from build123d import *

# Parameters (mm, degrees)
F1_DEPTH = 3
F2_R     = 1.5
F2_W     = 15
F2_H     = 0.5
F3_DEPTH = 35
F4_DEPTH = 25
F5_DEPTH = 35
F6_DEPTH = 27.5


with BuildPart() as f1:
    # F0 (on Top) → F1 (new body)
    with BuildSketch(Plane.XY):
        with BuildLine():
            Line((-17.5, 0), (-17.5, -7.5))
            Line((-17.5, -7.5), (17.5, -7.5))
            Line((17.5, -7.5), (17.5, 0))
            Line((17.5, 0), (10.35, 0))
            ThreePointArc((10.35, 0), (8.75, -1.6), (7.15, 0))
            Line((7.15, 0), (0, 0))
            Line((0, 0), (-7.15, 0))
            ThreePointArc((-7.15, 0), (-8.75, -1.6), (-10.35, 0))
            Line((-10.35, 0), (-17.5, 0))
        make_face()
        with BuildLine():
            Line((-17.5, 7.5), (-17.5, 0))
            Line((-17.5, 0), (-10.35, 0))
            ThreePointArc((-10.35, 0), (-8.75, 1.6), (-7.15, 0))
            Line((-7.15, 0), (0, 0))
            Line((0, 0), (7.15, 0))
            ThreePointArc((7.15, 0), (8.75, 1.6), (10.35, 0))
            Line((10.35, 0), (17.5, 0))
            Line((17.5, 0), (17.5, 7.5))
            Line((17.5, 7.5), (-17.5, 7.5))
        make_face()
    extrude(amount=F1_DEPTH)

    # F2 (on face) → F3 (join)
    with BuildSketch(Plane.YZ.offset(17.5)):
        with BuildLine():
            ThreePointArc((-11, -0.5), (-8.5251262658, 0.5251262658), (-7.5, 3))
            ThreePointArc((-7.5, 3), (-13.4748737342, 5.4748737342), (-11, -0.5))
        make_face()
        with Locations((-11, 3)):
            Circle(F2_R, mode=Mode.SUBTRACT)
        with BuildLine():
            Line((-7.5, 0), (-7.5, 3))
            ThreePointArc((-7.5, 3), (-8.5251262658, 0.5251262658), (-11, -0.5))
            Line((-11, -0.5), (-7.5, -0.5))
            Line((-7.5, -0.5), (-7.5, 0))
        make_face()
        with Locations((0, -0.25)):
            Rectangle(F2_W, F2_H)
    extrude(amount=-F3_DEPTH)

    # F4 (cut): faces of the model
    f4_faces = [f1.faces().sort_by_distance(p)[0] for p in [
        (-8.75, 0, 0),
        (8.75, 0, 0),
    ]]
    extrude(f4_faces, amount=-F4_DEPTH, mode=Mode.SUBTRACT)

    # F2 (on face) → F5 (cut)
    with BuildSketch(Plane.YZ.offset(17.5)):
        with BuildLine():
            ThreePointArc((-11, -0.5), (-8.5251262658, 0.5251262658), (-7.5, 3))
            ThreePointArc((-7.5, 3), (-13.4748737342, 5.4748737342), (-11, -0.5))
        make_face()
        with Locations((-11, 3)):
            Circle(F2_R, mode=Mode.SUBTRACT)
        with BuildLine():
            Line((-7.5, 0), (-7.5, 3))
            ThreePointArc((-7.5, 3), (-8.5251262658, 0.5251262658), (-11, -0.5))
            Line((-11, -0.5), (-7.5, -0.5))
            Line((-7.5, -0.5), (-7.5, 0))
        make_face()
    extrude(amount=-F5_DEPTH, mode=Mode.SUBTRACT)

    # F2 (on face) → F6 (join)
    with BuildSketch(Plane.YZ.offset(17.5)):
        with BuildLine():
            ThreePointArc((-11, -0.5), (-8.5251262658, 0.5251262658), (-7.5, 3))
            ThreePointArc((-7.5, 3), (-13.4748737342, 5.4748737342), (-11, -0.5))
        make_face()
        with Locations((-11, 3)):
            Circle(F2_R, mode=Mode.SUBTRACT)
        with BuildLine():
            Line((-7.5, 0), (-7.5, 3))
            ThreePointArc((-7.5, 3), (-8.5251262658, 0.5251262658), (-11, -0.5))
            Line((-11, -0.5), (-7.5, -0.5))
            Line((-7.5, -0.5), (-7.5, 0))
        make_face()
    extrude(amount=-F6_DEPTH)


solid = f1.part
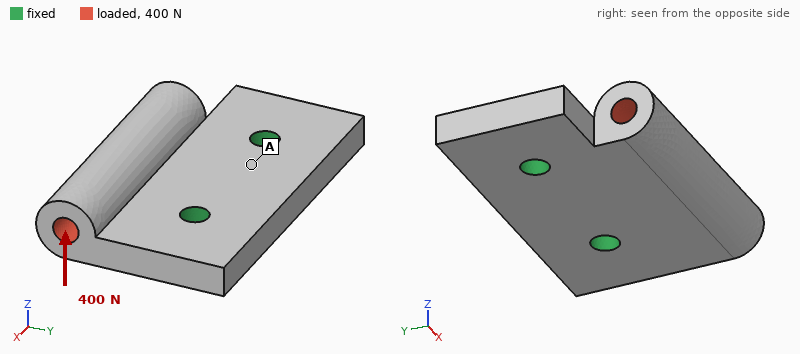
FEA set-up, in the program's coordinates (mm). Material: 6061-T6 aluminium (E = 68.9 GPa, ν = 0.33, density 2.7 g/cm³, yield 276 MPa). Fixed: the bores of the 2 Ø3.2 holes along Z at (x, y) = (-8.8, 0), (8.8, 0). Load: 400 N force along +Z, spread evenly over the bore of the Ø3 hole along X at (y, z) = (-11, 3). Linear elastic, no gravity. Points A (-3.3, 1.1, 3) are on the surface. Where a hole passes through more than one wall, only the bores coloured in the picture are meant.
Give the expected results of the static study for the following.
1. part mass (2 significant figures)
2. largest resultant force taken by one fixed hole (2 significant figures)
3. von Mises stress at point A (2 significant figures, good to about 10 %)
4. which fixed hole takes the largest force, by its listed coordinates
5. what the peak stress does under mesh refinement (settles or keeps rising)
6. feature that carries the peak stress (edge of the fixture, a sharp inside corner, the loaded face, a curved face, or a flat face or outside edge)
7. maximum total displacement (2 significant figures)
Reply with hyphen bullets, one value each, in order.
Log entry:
- 7.3 g
- 270 N
- 18 MPa
- (8.8, 0)
- keeps rising
- edge of the fixture
- 43 µm
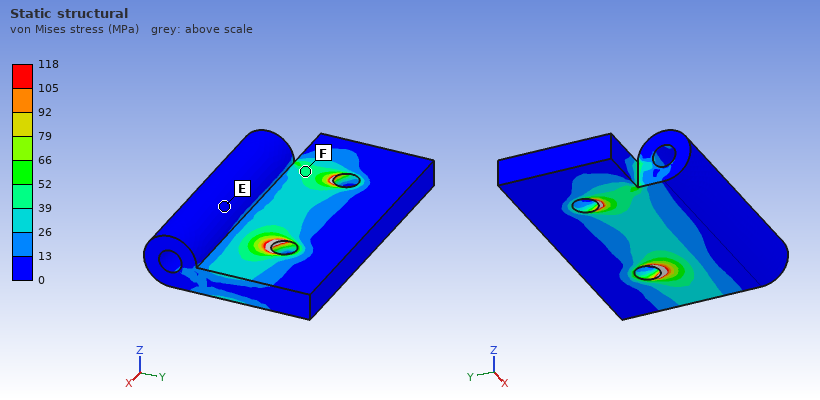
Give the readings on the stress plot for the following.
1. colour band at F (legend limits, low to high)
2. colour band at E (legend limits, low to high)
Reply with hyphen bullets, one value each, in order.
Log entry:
- 39 to 52 MPa
- 0 to 13 MPa
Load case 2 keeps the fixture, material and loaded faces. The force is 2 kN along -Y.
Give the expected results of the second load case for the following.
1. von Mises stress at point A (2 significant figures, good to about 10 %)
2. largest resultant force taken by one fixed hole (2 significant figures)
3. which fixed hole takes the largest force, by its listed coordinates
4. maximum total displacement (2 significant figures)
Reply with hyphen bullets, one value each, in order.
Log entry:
- 24 MPa
- 1.4 kN
- (8.8, 0)
- 50 µm
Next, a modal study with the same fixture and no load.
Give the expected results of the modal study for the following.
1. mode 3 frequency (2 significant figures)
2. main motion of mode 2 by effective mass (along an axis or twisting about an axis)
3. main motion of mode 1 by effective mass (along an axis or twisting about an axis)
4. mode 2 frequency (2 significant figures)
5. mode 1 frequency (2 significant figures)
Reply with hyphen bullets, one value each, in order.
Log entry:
- 33 kHz
- twisting about Y
- along Z
- 20 kHz
- 11 kHz
